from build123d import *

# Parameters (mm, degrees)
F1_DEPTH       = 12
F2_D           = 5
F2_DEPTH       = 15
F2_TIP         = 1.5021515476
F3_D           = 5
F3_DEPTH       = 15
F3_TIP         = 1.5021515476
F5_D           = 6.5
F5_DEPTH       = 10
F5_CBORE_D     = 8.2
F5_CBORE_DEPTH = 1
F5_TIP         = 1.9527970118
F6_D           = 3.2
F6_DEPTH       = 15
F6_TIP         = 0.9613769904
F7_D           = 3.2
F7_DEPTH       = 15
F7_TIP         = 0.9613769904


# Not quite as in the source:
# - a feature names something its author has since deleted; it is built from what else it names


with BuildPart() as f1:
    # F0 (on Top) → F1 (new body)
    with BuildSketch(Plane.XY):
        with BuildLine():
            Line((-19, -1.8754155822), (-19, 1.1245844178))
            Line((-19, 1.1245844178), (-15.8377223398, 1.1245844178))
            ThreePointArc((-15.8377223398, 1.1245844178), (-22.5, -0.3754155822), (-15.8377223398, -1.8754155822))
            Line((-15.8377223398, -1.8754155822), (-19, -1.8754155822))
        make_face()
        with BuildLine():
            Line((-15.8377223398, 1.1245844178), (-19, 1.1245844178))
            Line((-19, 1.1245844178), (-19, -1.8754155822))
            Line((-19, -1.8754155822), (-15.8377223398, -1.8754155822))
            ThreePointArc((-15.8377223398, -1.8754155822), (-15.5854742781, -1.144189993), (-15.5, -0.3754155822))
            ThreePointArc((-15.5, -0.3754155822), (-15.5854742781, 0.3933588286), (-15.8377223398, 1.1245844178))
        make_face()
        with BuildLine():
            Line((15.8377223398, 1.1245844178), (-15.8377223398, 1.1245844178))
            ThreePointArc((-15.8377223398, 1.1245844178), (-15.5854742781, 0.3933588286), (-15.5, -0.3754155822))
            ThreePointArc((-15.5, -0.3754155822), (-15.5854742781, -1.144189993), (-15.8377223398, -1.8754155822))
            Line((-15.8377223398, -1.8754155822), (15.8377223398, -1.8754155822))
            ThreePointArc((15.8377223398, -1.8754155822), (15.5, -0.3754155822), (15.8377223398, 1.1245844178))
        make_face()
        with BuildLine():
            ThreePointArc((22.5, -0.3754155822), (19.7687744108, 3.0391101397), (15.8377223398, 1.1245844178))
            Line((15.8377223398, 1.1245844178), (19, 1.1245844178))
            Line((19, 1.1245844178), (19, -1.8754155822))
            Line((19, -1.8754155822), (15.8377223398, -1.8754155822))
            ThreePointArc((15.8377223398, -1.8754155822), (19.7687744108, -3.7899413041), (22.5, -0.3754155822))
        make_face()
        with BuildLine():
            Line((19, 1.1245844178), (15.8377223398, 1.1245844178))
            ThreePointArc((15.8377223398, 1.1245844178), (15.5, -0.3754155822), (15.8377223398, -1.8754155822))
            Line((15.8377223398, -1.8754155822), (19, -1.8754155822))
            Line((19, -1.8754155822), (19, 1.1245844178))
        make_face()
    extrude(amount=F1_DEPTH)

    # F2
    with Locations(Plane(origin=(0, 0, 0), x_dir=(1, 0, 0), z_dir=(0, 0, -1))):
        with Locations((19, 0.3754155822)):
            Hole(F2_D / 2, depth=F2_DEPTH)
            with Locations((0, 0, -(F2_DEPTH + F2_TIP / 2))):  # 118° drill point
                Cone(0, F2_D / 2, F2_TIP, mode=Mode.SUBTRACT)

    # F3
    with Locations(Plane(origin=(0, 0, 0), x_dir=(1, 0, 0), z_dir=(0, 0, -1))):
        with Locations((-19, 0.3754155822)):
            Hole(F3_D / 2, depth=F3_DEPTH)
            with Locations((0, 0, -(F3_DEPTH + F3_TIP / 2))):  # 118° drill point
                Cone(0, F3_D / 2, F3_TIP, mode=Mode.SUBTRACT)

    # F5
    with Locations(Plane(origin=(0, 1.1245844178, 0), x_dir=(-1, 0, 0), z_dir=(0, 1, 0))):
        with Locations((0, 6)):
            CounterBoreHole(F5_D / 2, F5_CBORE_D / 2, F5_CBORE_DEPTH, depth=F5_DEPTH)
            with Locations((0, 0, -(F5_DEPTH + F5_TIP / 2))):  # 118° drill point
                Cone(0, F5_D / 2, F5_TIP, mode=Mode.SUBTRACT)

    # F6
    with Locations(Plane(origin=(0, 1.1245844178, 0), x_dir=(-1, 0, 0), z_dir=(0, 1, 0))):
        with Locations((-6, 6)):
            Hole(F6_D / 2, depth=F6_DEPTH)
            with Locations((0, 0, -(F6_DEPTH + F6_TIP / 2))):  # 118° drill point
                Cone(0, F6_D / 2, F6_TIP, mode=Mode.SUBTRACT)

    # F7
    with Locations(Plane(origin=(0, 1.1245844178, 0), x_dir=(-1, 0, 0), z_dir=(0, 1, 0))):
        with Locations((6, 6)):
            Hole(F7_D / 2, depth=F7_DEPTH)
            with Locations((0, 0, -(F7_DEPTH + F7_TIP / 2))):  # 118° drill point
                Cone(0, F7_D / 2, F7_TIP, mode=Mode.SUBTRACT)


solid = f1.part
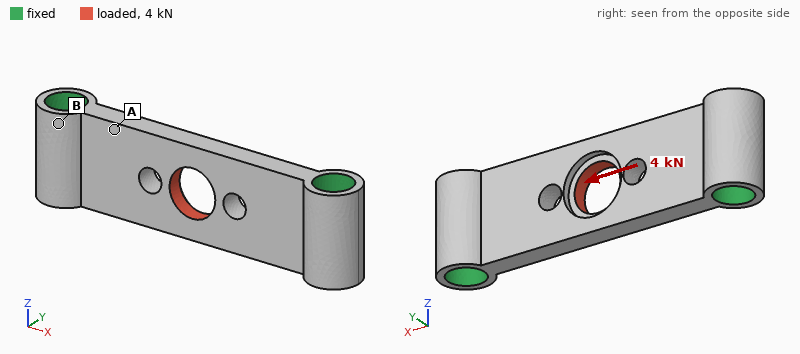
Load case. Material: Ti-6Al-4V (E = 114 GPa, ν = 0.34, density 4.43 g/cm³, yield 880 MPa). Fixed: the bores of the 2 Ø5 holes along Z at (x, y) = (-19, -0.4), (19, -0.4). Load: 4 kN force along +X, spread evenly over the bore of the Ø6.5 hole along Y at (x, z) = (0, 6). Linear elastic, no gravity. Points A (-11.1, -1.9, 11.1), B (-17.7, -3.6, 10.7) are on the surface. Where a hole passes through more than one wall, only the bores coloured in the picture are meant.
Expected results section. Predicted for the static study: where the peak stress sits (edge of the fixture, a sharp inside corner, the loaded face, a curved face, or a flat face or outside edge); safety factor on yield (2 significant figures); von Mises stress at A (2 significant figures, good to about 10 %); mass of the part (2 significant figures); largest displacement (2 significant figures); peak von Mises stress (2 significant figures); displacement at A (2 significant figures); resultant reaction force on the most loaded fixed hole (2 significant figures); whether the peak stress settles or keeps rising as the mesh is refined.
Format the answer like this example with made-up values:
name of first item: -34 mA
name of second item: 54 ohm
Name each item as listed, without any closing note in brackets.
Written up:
where the peak stress sits: a curved face
safety factor on yield: 2.8
von Mises stress at A: 66 MPa
mass of the part: 6.2 g
largest displacement: 14 µm
peak von Mises stress: 310 MPa
displacement at A: 2.9 µm
resultant reaction force on the most loaded fixed hole: 2.0 kN
whether the peak stress settles or keeps rising as the mesh is refined: settles
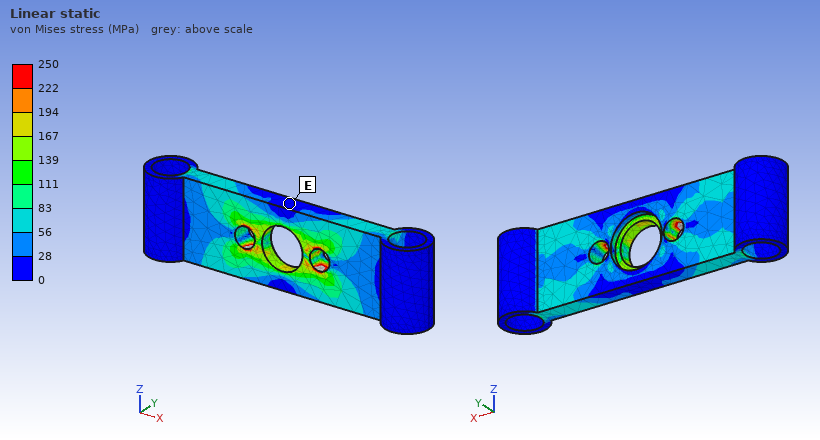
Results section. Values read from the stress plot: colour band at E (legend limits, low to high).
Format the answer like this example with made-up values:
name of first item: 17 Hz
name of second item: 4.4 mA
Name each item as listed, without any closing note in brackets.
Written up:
colour band at E: 0 to 28 MPa
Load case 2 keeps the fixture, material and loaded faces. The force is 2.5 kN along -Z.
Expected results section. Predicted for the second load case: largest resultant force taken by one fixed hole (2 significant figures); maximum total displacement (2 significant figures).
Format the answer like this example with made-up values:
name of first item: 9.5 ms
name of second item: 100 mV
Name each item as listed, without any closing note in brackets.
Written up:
largest resultant force taken by one fixed hole: 1.3 kN
maximum total displacement: 36 µm
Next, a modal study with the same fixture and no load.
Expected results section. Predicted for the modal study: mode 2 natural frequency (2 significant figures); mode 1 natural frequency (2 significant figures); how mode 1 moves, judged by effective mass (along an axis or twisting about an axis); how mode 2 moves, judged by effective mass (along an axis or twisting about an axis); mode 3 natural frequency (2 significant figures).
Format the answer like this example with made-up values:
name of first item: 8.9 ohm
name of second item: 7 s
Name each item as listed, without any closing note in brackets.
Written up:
mode 2 natural frequency: 24 kHz
mode 1 natural frequency: 15 kHz
how mode 1 moves, judged by effective mass: along Y
how mode 2 moves, judged by effective mass: twisting about X
mode 3 natural frequency: 35 kHz
